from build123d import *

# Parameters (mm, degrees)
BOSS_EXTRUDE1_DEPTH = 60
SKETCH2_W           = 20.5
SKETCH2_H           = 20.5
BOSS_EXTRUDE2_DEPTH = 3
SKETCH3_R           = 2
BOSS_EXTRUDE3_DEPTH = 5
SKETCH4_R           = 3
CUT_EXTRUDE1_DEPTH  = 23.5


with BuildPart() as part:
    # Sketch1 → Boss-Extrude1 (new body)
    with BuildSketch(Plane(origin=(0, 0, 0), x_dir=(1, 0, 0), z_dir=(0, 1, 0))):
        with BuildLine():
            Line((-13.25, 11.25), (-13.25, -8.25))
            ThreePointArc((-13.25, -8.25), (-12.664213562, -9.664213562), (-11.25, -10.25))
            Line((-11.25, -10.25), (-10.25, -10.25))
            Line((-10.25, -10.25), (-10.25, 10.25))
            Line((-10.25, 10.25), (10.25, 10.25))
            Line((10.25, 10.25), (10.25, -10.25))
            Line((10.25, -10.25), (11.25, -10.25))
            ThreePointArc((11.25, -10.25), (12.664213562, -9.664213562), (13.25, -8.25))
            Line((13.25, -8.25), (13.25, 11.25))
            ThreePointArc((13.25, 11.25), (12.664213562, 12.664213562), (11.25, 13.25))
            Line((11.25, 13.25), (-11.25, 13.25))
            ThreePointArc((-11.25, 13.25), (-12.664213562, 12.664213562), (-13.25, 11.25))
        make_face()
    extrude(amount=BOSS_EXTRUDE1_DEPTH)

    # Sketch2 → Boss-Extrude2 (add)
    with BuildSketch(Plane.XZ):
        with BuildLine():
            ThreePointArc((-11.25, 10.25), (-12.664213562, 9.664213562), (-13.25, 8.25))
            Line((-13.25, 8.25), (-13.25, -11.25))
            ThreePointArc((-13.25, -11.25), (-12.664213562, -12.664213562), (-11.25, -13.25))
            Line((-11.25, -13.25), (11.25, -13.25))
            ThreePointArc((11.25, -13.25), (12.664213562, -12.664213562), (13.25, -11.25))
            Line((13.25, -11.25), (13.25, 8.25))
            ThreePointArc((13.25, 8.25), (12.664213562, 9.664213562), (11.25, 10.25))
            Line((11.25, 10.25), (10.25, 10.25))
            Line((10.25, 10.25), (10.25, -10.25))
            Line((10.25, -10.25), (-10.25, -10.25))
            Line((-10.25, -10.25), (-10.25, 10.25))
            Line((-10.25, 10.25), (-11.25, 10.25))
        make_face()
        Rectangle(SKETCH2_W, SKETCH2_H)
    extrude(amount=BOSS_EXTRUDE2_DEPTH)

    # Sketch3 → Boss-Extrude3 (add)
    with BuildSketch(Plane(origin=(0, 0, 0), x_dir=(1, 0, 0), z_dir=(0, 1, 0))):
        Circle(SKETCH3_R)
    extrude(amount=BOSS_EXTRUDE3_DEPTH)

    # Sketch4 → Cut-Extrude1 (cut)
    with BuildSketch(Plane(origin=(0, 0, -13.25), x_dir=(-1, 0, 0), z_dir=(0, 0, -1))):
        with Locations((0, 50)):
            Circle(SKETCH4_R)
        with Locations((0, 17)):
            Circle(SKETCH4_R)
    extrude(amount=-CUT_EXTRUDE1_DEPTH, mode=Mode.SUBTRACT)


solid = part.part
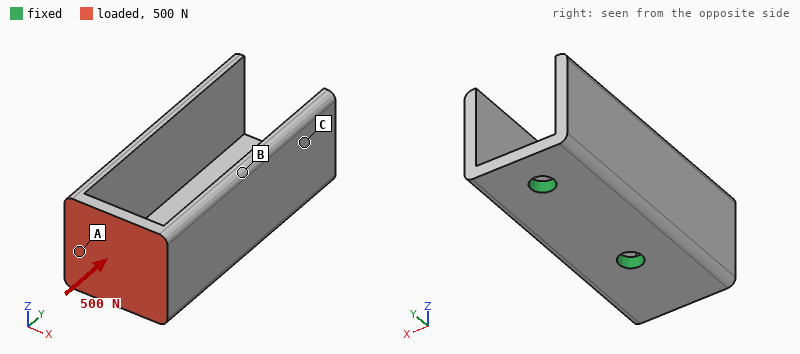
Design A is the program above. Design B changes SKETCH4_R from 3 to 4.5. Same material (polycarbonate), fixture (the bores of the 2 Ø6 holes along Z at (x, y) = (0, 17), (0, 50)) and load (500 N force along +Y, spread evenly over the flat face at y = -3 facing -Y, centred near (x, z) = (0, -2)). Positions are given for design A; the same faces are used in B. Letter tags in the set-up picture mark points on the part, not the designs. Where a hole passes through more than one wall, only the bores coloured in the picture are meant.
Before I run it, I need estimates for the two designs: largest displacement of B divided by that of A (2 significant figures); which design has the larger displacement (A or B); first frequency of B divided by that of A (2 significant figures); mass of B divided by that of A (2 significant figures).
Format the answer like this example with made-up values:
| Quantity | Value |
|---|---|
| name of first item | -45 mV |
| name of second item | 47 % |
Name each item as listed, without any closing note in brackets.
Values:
| Quantity | Value |
|---|---|
| largest displacement of B divided by that of A | 0.87 |
| which design has the larger displacement | A |
| first frequency of B divided by that of A | 1.2 |
| mass of B divided by that of A | 0.98 |
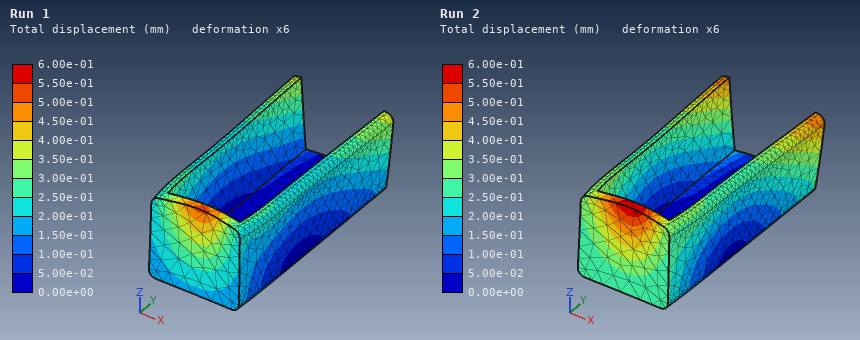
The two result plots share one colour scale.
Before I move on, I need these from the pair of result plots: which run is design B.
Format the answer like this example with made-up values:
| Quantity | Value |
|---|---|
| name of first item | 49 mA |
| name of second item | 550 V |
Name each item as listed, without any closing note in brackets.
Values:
| Quantity | Value |
|---|---|
| which run is design B | Run 1 |
